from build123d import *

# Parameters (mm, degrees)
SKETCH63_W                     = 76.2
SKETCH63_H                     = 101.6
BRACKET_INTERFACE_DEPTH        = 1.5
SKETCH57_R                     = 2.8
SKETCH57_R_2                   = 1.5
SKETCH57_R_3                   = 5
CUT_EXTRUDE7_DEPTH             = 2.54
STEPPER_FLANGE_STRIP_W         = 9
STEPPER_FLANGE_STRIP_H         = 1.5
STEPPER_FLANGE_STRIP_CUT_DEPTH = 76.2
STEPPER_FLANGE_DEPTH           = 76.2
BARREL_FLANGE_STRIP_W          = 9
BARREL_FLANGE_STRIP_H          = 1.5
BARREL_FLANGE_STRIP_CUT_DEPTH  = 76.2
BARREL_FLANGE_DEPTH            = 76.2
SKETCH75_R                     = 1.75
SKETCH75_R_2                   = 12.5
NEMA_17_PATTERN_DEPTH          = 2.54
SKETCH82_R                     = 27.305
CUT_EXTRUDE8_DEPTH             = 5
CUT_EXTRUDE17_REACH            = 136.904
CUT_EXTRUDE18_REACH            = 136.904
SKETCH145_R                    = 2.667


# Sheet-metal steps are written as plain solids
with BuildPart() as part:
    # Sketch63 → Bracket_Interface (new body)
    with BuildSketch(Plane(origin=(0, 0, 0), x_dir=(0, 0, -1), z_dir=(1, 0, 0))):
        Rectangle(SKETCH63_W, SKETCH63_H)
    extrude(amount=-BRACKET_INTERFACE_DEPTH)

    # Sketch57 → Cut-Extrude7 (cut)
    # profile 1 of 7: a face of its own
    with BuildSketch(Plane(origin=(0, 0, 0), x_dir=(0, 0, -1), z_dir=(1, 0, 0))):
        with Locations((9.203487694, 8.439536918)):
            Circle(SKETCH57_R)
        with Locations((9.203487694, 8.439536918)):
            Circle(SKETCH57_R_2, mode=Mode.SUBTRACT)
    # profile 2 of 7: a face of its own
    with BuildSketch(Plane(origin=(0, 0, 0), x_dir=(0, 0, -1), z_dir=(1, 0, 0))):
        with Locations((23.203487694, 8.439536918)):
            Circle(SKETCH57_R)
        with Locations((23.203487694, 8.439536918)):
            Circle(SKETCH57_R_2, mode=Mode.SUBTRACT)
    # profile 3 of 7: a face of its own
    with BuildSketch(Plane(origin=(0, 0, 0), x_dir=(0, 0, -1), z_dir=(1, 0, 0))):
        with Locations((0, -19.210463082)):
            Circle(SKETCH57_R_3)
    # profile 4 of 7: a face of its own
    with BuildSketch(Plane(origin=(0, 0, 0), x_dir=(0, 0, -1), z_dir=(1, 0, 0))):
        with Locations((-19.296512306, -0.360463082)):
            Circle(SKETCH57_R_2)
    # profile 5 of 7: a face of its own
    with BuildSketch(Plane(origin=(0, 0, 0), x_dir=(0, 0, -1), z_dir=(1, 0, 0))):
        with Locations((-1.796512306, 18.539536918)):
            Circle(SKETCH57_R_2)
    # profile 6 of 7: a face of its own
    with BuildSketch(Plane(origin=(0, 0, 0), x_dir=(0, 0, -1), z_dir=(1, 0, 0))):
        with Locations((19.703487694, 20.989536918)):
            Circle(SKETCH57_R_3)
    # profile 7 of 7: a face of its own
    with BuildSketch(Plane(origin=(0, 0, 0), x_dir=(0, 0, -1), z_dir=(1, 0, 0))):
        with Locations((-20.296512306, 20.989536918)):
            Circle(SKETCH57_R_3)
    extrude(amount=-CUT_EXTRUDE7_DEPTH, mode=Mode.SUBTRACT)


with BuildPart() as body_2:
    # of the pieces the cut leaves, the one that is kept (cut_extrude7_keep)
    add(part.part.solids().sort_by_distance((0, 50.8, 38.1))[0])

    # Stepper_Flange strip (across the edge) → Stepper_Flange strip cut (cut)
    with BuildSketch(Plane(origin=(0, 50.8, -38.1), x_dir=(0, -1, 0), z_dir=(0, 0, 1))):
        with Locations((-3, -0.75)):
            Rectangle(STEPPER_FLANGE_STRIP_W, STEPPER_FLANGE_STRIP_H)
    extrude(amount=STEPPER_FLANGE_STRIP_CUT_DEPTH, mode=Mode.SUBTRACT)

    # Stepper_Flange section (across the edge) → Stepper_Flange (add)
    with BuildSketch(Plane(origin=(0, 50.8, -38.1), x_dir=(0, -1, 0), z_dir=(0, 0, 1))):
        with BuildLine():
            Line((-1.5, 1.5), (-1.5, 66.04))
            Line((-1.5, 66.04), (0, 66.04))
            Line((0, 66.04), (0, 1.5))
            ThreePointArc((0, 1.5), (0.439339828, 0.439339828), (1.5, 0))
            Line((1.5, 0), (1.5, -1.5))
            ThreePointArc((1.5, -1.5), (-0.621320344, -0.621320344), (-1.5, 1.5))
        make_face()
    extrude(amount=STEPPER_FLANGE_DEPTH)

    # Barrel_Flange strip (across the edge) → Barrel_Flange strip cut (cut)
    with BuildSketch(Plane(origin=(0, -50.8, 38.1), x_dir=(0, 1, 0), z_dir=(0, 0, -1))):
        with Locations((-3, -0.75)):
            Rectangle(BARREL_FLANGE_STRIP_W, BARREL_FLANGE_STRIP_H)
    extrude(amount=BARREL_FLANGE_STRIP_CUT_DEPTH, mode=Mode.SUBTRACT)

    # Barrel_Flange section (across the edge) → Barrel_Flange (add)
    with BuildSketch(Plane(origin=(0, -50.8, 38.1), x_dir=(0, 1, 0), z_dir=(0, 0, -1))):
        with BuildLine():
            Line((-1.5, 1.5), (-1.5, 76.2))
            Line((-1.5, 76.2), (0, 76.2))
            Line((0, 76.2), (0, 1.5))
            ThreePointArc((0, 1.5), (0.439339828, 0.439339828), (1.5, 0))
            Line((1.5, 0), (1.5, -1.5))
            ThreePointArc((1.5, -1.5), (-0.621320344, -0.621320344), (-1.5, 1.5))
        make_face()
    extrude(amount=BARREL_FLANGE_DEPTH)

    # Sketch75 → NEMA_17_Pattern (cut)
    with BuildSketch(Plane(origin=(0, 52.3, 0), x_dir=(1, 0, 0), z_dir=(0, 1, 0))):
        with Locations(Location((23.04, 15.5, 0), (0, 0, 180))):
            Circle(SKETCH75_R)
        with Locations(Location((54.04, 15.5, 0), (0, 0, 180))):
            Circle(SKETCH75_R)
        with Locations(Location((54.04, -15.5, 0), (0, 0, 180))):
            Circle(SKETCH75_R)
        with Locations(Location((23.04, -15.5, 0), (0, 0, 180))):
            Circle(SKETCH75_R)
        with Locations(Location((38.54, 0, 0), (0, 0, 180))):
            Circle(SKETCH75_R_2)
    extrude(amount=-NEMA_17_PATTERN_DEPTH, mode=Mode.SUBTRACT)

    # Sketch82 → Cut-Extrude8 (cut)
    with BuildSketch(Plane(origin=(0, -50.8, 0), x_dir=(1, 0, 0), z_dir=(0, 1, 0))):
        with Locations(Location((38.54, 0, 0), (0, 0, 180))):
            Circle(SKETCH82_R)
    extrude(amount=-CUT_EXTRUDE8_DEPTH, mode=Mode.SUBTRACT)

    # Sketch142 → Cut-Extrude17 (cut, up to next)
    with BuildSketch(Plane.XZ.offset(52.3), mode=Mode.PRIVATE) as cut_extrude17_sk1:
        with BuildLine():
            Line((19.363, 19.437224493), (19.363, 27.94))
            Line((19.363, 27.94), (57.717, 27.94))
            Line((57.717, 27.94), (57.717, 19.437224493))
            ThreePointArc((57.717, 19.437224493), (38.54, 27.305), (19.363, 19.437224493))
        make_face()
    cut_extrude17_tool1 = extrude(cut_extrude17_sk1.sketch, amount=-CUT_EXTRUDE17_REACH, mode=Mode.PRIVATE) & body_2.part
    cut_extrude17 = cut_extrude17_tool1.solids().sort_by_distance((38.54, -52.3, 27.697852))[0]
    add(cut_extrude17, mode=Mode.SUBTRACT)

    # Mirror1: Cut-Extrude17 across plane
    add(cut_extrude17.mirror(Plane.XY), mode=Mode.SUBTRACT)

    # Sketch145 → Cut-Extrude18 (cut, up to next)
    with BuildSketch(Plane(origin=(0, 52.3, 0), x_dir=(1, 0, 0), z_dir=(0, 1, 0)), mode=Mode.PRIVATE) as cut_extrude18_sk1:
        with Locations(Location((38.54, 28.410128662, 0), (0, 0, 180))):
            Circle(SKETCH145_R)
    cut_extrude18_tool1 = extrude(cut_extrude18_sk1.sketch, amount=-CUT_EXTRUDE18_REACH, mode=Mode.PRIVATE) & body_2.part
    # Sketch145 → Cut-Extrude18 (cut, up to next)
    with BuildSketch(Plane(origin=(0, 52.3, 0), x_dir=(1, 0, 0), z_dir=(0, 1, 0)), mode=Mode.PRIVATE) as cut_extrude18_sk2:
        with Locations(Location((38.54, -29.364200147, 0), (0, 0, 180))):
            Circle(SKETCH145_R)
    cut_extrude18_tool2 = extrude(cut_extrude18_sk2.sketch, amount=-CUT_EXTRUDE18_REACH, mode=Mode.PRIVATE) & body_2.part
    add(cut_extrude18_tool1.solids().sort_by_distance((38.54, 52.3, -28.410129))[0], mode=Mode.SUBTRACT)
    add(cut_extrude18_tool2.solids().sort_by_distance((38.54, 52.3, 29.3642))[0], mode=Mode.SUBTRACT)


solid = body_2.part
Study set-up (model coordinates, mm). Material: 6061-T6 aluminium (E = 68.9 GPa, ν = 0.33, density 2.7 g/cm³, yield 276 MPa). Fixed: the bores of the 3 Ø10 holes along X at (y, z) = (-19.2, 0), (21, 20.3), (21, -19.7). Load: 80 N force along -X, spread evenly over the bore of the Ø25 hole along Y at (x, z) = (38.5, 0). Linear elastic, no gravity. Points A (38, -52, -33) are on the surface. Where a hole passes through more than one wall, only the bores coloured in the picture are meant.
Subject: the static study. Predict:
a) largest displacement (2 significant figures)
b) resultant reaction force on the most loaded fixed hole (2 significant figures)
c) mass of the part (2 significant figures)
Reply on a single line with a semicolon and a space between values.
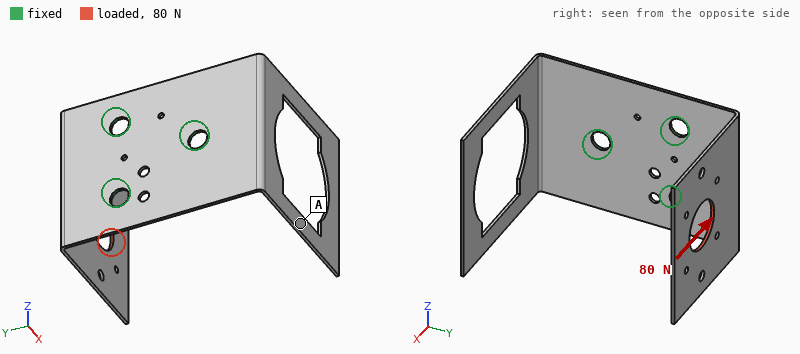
1.3 mm; 42 N; 62 g
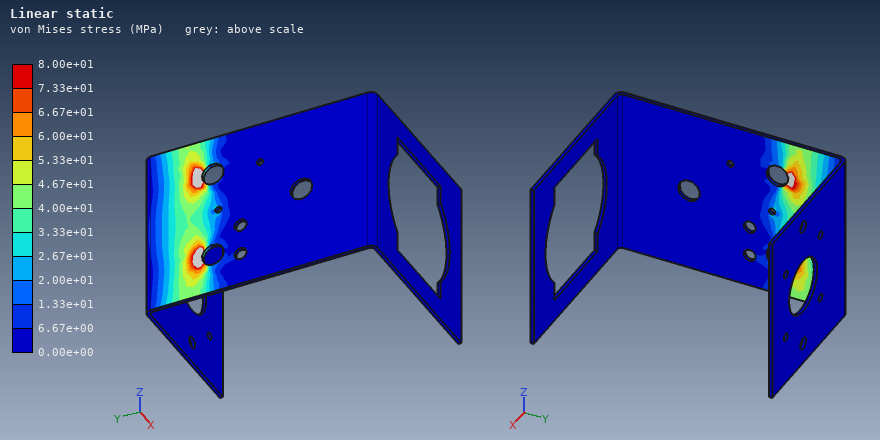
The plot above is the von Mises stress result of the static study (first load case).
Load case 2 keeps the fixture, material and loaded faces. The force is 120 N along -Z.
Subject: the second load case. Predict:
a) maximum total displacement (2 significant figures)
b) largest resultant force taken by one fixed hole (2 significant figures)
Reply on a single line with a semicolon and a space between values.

1.5 mm; 130 N
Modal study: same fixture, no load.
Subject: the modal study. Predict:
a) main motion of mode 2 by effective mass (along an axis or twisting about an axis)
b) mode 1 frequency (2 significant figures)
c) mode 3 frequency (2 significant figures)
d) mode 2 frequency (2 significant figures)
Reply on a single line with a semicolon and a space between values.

along Y; 130 Hz; 230 Hz; 180 Hz
